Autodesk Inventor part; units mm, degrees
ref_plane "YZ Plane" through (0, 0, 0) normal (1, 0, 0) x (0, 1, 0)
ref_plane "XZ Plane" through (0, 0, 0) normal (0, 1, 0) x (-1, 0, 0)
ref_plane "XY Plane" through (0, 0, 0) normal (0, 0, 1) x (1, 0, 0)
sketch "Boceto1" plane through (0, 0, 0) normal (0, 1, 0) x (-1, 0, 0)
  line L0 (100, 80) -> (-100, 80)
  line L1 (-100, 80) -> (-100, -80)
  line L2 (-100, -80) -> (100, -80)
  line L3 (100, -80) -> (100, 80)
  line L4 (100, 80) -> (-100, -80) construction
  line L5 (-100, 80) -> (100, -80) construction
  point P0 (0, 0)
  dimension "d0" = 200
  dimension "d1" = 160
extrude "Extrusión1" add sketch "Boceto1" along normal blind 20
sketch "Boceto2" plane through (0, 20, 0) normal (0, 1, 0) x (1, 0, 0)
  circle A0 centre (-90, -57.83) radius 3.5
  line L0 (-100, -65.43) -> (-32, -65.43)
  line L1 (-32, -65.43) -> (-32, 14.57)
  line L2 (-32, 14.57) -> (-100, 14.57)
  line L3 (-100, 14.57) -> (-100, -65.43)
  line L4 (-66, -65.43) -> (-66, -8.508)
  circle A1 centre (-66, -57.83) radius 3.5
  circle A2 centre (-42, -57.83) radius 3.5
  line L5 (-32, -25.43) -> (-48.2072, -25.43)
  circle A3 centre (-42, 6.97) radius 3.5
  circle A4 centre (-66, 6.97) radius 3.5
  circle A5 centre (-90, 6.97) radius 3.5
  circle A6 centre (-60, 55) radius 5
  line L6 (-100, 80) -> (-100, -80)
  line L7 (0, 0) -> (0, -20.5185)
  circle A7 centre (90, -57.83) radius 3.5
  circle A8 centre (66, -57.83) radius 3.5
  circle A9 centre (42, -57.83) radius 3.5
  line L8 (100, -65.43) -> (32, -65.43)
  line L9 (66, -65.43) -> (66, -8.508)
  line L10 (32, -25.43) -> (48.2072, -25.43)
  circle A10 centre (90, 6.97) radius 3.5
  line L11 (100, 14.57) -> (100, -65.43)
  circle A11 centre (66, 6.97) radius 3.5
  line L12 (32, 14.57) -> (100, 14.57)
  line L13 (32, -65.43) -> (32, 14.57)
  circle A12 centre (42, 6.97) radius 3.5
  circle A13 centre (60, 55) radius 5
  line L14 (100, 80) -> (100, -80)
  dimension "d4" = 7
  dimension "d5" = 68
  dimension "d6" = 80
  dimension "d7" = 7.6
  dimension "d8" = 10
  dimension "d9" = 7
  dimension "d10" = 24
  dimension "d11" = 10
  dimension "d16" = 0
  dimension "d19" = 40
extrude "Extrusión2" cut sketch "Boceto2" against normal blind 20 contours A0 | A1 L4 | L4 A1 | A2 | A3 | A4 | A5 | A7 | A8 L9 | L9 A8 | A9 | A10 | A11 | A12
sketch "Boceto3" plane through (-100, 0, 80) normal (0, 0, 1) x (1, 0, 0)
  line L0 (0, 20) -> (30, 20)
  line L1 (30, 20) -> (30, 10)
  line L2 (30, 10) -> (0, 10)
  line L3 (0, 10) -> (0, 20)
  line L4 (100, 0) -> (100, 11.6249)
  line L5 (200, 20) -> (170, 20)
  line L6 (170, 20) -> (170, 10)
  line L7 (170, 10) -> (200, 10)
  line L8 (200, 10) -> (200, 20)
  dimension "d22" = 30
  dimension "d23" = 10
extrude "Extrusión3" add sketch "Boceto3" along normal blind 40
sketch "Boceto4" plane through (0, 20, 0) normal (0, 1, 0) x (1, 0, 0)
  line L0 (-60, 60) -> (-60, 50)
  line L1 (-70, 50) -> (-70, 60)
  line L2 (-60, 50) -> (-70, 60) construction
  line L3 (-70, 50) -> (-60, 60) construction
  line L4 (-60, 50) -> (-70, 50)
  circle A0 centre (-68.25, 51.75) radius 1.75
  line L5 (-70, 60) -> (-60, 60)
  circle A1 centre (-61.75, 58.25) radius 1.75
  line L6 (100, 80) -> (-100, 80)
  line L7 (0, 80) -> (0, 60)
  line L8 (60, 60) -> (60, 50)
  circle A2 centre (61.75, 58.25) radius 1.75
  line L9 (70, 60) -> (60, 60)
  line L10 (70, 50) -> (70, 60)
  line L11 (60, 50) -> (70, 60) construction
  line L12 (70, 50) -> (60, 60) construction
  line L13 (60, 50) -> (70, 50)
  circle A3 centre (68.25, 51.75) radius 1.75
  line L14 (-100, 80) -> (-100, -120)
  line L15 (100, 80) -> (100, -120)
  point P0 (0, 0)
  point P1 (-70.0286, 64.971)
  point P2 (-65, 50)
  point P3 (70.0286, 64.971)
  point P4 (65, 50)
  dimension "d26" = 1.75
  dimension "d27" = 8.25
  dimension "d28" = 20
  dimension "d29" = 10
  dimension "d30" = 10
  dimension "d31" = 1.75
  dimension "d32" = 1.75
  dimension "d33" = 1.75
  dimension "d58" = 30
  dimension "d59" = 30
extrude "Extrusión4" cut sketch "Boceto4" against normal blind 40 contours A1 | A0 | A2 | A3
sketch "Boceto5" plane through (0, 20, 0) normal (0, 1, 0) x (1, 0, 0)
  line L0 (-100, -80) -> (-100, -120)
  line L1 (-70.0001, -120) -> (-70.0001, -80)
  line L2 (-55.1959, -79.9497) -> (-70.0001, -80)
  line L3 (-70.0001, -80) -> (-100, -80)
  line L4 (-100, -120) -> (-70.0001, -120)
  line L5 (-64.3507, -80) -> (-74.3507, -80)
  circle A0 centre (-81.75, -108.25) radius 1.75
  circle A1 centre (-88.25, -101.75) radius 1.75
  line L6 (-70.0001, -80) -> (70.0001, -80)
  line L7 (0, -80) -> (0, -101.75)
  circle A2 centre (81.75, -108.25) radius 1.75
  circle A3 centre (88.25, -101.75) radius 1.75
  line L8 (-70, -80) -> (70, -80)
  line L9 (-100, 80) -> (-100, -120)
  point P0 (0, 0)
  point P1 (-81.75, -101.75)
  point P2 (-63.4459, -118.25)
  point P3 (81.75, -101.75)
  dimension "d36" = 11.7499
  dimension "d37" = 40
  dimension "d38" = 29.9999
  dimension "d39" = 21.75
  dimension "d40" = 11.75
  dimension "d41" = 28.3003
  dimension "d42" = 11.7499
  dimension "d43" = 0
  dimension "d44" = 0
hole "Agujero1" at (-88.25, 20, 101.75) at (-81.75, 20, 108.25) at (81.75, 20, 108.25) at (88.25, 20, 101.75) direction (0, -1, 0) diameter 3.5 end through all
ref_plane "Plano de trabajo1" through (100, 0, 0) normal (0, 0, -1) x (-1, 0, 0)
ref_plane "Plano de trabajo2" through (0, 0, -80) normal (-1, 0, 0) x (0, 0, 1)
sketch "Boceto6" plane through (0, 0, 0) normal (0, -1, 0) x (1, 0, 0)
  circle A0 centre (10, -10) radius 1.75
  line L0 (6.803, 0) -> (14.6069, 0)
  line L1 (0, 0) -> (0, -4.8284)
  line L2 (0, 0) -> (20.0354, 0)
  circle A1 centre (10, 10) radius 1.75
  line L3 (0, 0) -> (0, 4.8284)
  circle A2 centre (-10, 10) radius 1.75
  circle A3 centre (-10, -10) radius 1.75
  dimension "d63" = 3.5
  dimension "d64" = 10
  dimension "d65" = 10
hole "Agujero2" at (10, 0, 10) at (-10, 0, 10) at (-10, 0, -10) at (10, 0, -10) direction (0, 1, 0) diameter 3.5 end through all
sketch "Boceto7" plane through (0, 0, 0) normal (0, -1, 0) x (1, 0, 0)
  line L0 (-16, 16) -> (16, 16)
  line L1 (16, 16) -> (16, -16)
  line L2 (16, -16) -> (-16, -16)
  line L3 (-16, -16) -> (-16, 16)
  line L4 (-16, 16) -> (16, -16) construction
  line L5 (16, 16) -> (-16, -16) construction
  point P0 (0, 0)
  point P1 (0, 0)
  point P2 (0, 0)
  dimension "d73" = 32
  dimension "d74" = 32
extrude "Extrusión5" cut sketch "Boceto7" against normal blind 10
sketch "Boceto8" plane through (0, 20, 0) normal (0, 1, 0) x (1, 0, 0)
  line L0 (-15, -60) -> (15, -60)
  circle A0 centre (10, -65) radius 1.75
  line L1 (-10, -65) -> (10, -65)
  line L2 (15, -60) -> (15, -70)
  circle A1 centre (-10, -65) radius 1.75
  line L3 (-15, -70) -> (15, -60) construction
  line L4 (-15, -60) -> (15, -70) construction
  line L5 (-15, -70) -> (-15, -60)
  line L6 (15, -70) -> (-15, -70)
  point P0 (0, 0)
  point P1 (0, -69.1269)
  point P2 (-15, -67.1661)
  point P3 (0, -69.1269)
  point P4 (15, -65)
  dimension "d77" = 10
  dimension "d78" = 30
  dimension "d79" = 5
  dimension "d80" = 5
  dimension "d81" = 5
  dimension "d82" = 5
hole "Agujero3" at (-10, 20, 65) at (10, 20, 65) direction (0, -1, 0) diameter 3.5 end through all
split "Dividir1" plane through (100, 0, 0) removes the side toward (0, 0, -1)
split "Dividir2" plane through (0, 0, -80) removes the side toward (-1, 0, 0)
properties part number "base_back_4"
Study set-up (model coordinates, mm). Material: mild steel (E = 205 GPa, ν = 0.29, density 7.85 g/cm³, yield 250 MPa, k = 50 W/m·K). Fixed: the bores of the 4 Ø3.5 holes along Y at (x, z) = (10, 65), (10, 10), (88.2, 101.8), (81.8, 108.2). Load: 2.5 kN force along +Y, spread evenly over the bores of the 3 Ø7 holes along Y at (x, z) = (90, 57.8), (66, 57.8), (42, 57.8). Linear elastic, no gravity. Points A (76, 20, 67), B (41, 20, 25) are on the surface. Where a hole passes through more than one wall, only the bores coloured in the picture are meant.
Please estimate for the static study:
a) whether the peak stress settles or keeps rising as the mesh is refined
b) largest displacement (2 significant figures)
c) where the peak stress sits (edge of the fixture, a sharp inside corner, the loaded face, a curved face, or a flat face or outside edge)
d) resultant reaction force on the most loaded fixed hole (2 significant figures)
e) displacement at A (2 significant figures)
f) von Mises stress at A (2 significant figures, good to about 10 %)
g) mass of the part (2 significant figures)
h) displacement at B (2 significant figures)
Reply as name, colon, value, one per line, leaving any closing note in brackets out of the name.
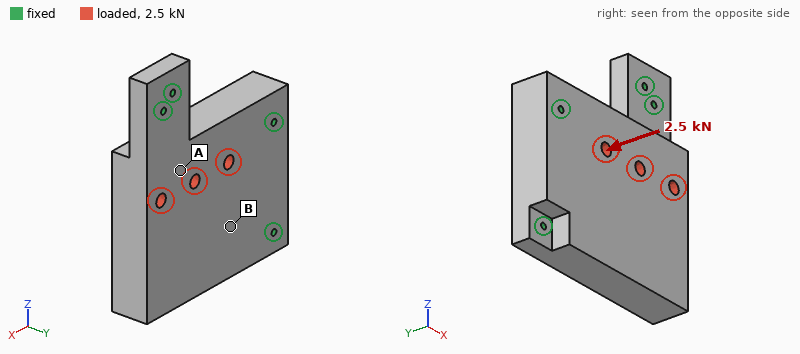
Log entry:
whether the peak stress settles or keeps rising as the mesh is refined: keeps rising
largest displacement: 22 µm
where the peak stress sits: edge of the fixture
resultant reaction force on the most loaded fixed hole: 1.5 kN
displacement at A: 9.9 µm
von Mises stress at A: 8.6 MPa
mass of the part: 1.3 kg
displacement at B: 6.6 µm
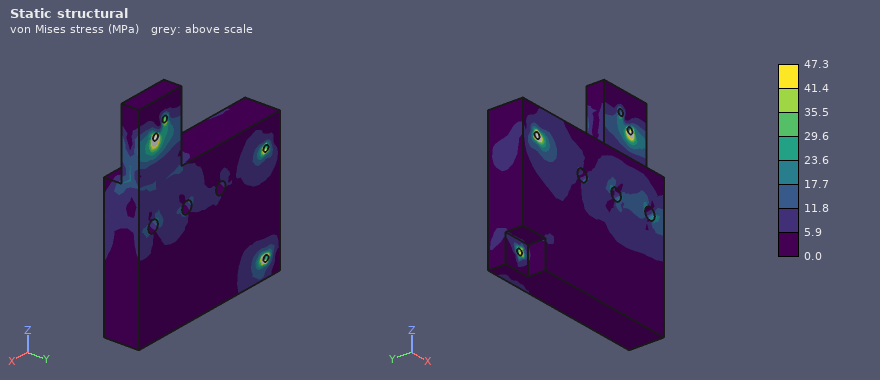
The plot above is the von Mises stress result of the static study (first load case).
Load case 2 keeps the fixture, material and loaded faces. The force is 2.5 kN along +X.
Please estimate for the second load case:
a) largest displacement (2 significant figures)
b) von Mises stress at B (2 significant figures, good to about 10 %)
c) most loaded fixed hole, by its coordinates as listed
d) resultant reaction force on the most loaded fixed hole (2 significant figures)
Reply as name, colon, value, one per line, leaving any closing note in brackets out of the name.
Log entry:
largest displacement: 1.4 µm
von Mises stress at B: 1.1 MPa
most loaded fixed hole, by its coordinates as listed: (10, 65)
resultant reaction force on the most loaded fixed hole: 1.7 kN
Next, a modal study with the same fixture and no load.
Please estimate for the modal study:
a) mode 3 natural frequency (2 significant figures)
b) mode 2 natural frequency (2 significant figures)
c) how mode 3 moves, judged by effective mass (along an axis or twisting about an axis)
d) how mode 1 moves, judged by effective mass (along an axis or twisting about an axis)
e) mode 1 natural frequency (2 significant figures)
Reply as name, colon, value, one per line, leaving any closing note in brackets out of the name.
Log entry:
mode 3 natural frequency: 7900 Hz
mode 2 natural frequency: 6600 Hz
how mode 3 moves, judged by effective mass: along Z
how mode 1 moves, judged by effective mass: along Y
mode 1 natural frequency: 2000 Hz
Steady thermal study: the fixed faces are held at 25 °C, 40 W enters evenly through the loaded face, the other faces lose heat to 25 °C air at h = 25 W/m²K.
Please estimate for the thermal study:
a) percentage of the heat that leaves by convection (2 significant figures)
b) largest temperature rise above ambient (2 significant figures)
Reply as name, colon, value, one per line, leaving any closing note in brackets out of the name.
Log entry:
percentage of the heat that leaves by convection: 20 %
largest temperature rise above ambient: 24 K
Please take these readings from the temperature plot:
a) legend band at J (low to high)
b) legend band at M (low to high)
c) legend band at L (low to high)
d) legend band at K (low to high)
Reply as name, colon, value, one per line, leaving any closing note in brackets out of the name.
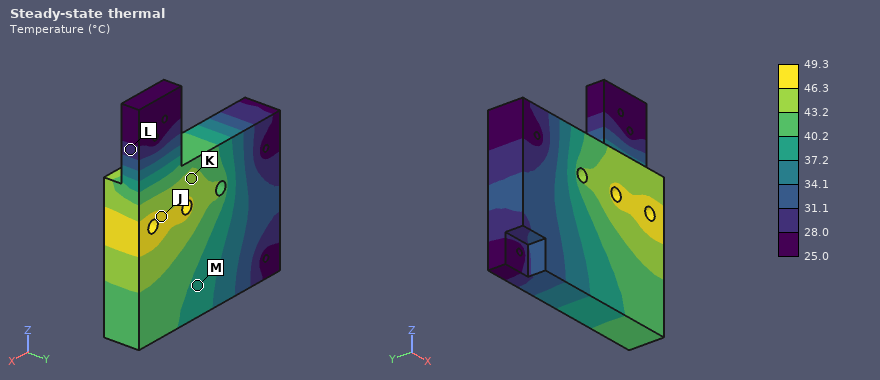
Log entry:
legend band at J: 46.3 to 49.3 °C
legend band at M: 37.2 to 40.2 °C
legend band at L: 28.0 to 31.1 °C
legend band at K: 43.2 to 46.3 °C
